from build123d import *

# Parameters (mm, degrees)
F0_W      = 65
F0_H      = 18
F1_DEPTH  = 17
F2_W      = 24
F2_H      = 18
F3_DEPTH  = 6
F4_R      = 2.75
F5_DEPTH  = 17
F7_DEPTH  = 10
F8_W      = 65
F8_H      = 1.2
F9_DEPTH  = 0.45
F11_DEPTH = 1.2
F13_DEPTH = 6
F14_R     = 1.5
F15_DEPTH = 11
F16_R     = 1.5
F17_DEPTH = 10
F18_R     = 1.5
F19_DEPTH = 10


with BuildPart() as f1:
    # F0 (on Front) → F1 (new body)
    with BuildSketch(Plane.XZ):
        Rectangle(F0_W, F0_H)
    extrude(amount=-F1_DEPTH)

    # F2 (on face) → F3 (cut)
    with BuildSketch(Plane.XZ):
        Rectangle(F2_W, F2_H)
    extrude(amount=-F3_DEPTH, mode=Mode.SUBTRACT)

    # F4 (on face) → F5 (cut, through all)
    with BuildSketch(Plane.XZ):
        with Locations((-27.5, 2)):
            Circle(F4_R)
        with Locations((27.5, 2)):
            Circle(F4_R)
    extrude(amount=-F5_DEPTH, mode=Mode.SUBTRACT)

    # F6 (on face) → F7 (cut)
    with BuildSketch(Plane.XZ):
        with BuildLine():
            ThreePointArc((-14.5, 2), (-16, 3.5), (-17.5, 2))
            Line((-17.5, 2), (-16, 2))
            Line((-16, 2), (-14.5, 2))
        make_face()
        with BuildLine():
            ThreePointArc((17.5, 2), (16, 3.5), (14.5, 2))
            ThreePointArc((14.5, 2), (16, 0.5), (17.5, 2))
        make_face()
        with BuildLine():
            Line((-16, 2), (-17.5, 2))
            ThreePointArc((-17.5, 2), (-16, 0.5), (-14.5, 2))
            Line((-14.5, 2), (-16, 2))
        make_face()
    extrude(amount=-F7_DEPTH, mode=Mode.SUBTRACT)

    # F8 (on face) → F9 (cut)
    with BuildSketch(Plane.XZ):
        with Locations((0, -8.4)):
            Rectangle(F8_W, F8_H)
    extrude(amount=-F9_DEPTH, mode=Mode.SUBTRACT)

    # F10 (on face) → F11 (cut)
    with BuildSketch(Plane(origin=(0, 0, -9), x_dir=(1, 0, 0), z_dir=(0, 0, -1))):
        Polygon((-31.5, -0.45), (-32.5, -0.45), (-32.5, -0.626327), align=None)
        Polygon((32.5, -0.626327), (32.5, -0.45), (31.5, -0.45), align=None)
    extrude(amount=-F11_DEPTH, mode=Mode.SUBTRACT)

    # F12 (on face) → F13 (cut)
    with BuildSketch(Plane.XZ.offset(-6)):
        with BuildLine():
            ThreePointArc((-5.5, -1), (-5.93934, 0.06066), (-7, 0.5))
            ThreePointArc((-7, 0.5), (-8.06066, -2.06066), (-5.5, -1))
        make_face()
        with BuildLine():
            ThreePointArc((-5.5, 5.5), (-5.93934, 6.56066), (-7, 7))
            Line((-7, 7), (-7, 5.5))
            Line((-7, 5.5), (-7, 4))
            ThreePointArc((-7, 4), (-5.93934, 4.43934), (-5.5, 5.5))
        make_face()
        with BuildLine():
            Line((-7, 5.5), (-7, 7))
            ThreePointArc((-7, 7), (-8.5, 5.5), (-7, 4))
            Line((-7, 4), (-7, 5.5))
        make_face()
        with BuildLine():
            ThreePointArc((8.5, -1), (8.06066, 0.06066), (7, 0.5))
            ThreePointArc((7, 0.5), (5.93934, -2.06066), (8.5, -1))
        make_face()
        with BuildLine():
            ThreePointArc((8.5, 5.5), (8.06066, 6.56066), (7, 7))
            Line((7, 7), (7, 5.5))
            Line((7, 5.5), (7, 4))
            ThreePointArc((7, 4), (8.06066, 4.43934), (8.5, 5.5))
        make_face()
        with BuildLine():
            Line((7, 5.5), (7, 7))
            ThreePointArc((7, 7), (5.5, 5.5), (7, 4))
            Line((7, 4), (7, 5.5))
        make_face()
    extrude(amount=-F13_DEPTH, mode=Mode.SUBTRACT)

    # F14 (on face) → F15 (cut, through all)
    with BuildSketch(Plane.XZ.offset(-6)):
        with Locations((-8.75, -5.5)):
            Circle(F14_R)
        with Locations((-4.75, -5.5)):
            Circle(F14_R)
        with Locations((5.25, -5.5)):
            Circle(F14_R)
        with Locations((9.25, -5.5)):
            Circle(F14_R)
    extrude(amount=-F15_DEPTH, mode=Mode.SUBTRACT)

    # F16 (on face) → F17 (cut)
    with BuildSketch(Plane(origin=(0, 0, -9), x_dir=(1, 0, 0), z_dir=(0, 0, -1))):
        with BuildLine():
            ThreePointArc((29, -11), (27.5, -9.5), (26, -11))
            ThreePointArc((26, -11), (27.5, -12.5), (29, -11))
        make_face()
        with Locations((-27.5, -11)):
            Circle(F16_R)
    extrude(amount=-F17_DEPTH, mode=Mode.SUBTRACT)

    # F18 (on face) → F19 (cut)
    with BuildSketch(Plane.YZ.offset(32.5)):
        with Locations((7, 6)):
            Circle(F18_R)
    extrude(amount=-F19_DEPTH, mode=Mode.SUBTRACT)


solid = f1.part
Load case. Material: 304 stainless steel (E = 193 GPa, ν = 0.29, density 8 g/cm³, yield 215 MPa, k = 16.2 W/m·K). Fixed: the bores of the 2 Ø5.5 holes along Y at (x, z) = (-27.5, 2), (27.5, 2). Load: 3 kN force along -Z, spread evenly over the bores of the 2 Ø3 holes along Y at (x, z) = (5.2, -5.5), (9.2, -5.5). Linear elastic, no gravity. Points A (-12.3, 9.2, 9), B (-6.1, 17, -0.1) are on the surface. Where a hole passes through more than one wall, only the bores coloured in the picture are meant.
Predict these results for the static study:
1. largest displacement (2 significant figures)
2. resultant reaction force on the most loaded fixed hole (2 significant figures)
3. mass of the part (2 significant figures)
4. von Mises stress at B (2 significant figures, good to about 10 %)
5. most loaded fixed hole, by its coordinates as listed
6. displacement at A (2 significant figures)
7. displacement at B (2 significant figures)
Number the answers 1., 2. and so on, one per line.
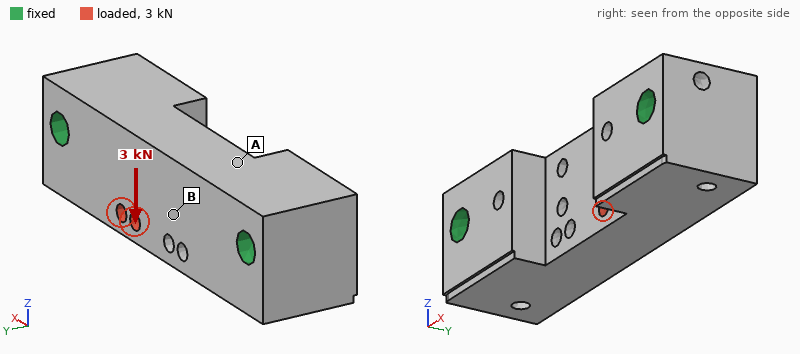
1. 7.2 µm
2. 2.0 kN
3. 130 g
4. 19 MPa
5. (27.5, 2)
6. 3.1 µm
7. 4.8 µm
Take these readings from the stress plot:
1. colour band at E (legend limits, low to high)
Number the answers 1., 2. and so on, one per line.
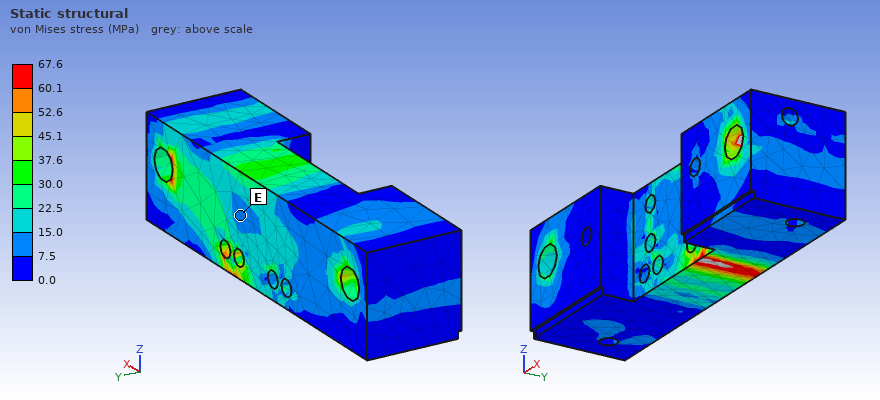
1. 7.5 to 15.0 MPa
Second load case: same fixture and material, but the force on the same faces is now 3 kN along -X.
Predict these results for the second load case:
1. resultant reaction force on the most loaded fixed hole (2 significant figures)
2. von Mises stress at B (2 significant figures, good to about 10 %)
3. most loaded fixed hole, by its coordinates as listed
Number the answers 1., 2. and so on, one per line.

1. 1.9 kN
2. 7.8 MPa
3. (27.5, 2)
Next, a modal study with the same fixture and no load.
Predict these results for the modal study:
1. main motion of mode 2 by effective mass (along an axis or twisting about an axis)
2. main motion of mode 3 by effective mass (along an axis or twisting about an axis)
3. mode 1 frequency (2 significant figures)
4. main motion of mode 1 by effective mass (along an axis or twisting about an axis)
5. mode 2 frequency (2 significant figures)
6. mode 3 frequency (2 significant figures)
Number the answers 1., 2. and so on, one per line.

1. along Y
2. twisting about X
3. 17 kHz
4. along Z
5. 20 kHz
6. 30 kHz
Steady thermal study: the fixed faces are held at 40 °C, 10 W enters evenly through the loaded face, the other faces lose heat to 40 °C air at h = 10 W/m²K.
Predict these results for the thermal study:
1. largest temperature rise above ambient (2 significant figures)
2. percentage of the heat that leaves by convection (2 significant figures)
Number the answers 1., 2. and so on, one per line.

1. 49 K
2. 6.4 %
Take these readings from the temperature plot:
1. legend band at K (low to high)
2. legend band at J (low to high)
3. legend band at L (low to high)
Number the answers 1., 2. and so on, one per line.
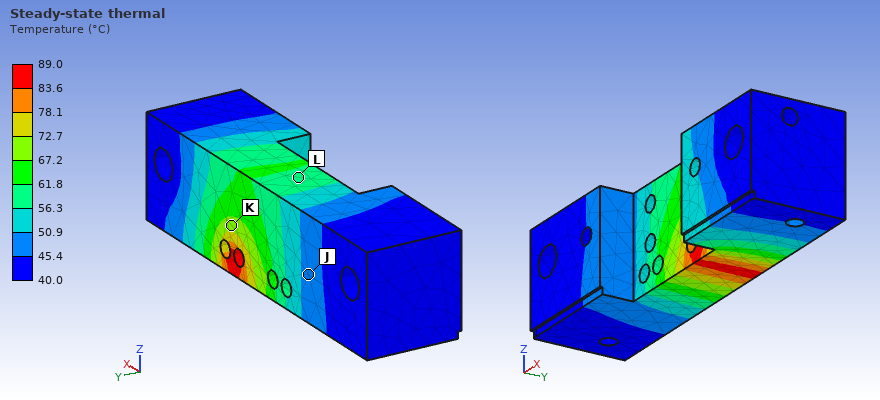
1. 67.2 to 72.7 °C
2. 45.4 to 50.9 °C
3. 56.3 to 61.8 °C
